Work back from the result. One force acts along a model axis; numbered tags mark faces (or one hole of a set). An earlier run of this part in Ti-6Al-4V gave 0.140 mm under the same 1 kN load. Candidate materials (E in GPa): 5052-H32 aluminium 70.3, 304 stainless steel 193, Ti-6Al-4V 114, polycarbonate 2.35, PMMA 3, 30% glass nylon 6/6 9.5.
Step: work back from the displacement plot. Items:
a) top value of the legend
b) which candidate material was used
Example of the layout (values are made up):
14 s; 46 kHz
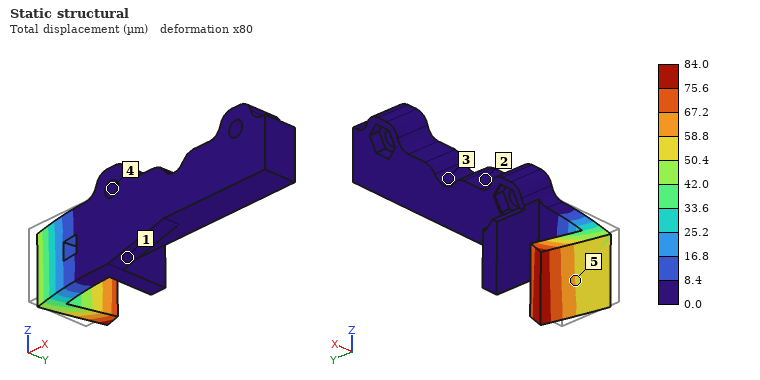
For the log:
84.0 µm; 304 stainless steel
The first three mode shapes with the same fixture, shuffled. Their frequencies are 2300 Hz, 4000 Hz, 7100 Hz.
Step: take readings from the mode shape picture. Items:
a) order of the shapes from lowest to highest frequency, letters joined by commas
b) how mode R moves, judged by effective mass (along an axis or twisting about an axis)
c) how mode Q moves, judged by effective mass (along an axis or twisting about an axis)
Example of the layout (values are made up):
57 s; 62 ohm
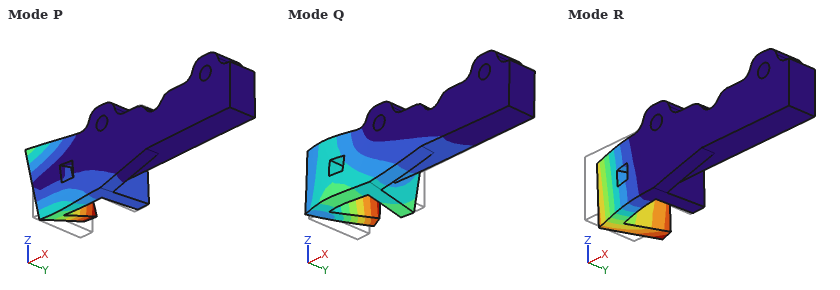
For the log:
R, P, Q; along Y; along Y
